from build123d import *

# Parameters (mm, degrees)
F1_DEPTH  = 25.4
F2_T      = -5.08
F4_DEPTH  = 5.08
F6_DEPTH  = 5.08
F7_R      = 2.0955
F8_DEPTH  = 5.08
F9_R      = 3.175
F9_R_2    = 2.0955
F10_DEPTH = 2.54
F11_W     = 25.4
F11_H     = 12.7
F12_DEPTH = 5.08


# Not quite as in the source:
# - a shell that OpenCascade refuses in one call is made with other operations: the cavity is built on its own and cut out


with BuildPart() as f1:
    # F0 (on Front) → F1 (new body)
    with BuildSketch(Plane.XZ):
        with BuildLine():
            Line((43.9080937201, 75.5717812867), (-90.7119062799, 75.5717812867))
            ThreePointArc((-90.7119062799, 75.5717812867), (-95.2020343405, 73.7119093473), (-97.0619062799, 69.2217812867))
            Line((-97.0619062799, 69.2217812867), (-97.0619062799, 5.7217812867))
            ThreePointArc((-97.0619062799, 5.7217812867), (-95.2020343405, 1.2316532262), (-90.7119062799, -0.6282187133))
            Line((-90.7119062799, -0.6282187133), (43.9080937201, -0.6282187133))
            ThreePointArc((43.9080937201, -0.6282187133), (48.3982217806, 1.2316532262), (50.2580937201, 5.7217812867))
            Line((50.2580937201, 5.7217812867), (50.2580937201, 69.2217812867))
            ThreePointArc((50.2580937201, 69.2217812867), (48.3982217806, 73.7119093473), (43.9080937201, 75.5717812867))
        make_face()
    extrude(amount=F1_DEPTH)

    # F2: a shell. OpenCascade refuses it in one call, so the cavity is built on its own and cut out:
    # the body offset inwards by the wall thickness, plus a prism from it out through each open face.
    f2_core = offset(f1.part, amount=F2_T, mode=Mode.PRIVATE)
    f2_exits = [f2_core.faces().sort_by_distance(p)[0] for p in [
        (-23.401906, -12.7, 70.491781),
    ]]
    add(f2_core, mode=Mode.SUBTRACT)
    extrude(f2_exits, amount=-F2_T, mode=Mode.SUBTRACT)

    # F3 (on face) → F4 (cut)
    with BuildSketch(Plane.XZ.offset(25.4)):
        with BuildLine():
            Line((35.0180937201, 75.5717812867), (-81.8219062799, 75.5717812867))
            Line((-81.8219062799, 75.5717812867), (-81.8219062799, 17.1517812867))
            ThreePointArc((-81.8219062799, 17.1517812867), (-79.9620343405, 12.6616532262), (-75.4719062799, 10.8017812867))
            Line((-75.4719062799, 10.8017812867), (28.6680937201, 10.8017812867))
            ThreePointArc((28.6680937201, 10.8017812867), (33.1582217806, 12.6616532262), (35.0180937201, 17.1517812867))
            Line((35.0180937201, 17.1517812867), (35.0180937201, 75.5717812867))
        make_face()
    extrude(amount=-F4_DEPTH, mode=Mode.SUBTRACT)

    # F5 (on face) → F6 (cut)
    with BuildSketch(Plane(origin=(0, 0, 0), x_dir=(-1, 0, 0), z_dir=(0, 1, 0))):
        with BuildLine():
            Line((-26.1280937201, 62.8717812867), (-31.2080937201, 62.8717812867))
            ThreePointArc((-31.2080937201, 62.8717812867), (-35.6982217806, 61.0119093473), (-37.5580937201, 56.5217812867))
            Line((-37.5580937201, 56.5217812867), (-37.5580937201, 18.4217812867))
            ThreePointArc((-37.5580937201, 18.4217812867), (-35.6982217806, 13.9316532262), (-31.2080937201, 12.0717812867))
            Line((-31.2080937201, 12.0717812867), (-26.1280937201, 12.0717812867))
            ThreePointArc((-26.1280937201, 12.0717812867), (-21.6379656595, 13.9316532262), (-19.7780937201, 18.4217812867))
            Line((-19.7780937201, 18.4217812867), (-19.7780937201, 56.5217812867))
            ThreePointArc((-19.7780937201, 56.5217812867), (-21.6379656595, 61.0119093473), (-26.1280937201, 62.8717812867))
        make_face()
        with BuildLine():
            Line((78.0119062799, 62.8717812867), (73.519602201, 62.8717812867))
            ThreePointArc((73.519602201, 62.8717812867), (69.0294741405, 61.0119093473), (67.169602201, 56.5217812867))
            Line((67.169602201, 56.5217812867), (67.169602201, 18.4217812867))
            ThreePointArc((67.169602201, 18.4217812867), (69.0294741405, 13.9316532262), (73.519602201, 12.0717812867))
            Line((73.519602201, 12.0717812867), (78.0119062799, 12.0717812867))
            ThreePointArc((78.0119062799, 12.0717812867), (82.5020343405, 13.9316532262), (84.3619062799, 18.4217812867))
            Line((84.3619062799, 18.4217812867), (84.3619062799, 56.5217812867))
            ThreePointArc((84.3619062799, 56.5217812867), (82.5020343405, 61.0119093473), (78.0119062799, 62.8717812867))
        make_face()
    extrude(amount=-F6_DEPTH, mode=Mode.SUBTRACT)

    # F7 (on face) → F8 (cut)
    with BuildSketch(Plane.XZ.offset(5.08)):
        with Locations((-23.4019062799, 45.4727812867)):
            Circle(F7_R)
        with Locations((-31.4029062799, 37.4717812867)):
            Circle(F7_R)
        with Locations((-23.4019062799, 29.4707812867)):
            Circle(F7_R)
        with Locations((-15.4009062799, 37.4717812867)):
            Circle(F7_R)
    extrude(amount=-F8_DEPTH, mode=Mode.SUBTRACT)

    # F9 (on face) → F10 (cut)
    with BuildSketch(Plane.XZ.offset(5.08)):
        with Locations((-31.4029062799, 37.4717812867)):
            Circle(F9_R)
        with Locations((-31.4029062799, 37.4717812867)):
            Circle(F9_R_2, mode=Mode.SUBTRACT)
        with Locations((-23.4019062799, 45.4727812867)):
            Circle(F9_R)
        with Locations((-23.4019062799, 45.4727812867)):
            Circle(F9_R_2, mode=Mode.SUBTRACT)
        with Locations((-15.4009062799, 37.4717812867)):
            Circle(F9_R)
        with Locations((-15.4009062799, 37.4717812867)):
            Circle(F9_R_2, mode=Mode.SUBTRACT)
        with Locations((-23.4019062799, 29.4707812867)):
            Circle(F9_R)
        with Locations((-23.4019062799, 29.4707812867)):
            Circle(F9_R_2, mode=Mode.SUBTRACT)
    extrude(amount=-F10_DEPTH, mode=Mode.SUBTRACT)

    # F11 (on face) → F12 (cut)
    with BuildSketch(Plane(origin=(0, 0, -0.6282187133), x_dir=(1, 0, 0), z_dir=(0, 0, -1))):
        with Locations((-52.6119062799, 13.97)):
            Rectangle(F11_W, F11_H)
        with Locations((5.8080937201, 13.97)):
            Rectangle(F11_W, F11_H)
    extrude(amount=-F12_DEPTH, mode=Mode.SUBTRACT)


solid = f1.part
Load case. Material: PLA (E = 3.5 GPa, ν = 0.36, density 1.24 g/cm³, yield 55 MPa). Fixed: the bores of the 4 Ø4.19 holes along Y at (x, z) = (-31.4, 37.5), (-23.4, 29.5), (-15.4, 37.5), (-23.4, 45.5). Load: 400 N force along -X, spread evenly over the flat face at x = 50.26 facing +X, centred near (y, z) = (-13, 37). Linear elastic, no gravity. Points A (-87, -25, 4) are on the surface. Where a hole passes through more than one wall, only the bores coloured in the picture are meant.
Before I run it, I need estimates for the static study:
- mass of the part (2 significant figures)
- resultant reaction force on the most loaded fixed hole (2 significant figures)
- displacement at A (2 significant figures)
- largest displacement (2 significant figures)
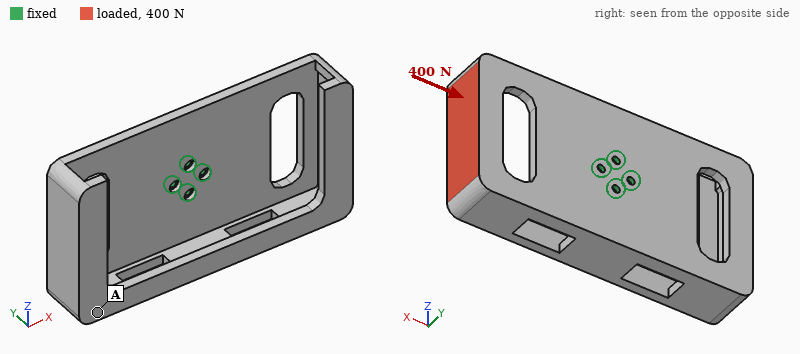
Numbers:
110 g
220 N
1.6 mm
1.8 mm
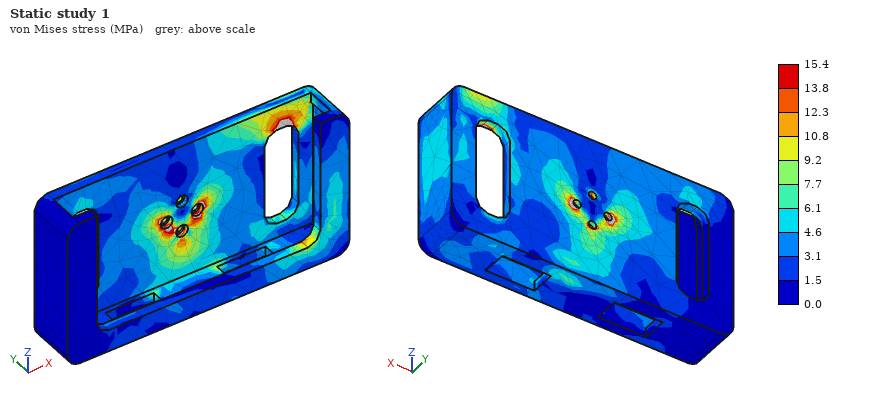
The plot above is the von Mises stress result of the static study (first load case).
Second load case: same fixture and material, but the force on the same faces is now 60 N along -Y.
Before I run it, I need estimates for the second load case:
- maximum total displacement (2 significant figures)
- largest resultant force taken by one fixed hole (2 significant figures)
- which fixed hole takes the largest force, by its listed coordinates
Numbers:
1.7 mm
230 N
(-15.4, 37.5)
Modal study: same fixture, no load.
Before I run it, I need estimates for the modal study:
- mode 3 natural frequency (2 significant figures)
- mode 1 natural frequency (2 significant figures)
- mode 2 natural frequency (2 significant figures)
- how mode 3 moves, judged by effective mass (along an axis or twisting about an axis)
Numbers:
350 Hz
160 Hz
280 Hz
along Y
